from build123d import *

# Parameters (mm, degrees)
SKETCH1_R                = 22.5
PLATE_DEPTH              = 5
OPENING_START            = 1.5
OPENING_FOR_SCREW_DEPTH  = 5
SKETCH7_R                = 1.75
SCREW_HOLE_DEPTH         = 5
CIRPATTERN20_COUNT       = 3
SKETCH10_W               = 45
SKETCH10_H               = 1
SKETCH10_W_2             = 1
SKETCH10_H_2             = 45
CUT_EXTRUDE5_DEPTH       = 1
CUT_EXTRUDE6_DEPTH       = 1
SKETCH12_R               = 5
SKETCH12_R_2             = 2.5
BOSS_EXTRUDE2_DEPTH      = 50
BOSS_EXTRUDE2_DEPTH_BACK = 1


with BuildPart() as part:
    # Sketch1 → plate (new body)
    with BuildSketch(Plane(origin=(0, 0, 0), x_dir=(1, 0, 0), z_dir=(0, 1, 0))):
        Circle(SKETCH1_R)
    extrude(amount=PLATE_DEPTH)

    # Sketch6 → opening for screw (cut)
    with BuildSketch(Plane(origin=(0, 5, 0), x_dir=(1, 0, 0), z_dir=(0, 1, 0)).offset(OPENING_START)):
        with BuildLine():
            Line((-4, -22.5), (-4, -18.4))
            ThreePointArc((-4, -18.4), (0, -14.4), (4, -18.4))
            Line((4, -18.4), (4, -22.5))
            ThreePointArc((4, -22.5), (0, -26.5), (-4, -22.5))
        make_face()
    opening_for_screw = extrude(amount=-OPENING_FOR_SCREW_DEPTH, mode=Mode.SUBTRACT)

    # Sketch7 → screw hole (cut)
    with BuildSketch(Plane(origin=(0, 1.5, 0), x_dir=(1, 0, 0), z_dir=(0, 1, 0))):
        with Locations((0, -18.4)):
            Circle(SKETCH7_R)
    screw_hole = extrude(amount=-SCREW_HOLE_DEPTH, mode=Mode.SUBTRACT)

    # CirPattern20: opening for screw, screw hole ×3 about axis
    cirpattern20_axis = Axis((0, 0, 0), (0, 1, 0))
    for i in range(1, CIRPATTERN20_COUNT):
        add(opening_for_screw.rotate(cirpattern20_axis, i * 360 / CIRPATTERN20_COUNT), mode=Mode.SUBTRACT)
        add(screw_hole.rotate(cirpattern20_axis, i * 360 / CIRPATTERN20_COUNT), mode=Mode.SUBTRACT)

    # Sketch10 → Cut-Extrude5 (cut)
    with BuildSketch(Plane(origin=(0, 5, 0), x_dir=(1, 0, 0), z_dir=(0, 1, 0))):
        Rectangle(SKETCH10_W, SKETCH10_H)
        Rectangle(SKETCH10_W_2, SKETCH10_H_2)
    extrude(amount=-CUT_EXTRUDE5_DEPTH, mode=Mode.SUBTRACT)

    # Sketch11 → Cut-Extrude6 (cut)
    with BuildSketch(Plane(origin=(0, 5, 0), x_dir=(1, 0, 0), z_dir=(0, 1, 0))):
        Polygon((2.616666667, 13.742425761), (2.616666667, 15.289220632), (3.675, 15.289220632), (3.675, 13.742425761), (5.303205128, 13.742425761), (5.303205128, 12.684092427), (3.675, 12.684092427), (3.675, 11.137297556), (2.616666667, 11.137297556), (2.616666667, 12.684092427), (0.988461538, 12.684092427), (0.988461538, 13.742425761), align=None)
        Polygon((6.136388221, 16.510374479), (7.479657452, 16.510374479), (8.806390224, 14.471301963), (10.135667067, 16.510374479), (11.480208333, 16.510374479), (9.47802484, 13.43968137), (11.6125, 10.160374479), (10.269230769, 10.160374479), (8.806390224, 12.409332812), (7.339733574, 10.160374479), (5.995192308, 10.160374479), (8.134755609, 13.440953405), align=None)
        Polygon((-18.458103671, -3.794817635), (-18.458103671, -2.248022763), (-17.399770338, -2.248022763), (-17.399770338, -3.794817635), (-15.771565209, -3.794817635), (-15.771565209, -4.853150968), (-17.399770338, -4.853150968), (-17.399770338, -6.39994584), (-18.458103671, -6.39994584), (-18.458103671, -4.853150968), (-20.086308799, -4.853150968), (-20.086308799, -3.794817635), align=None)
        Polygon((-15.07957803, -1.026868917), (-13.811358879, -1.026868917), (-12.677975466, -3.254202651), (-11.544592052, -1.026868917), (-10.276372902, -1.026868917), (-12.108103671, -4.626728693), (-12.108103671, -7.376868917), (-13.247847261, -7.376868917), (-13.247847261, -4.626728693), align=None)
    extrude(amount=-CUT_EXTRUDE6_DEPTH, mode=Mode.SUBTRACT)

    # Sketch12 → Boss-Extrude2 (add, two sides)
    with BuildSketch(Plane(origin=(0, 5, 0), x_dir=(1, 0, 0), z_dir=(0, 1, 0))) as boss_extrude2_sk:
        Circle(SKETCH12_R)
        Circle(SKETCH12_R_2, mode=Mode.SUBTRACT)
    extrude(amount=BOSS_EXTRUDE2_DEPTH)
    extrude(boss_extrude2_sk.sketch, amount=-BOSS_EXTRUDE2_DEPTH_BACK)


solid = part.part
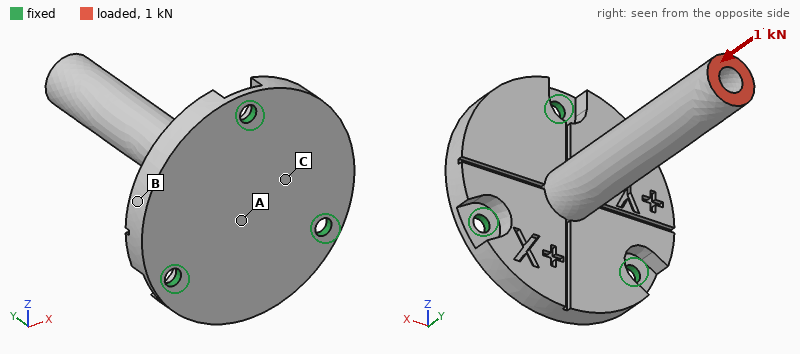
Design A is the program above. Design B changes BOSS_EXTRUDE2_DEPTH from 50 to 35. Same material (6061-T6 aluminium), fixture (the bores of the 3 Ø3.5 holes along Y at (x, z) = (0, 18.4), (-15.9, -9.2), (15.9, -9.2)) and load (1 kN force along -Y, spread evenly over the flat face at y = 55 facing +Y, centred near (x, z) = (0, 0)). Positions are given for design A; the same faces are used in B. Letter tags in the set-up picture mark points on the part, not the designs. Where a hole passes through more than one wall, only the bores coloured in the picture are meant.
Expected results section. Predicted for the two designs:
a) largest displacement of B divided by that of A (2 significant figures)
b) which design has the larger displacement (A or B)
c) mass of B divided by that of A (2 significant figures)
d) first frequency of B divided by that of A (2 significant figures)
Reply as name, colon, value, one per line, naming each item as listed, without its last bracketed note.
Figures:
largest displacement of B divided by that of A: 0.88
which design has the larger displacement: A
mass of B divided by that of A: 0.91
first frequency of B divided by that of A: 1.8
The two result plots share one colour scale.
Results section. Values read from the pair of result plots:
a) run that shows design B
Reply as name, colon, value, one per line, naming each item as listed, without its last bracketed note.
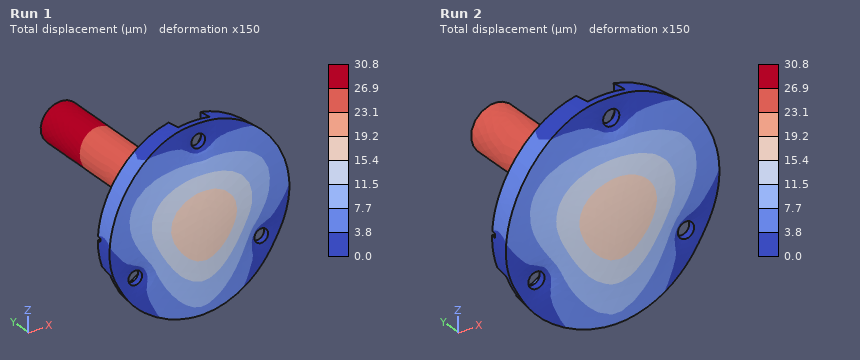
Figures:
run that shows design B: Run 2
